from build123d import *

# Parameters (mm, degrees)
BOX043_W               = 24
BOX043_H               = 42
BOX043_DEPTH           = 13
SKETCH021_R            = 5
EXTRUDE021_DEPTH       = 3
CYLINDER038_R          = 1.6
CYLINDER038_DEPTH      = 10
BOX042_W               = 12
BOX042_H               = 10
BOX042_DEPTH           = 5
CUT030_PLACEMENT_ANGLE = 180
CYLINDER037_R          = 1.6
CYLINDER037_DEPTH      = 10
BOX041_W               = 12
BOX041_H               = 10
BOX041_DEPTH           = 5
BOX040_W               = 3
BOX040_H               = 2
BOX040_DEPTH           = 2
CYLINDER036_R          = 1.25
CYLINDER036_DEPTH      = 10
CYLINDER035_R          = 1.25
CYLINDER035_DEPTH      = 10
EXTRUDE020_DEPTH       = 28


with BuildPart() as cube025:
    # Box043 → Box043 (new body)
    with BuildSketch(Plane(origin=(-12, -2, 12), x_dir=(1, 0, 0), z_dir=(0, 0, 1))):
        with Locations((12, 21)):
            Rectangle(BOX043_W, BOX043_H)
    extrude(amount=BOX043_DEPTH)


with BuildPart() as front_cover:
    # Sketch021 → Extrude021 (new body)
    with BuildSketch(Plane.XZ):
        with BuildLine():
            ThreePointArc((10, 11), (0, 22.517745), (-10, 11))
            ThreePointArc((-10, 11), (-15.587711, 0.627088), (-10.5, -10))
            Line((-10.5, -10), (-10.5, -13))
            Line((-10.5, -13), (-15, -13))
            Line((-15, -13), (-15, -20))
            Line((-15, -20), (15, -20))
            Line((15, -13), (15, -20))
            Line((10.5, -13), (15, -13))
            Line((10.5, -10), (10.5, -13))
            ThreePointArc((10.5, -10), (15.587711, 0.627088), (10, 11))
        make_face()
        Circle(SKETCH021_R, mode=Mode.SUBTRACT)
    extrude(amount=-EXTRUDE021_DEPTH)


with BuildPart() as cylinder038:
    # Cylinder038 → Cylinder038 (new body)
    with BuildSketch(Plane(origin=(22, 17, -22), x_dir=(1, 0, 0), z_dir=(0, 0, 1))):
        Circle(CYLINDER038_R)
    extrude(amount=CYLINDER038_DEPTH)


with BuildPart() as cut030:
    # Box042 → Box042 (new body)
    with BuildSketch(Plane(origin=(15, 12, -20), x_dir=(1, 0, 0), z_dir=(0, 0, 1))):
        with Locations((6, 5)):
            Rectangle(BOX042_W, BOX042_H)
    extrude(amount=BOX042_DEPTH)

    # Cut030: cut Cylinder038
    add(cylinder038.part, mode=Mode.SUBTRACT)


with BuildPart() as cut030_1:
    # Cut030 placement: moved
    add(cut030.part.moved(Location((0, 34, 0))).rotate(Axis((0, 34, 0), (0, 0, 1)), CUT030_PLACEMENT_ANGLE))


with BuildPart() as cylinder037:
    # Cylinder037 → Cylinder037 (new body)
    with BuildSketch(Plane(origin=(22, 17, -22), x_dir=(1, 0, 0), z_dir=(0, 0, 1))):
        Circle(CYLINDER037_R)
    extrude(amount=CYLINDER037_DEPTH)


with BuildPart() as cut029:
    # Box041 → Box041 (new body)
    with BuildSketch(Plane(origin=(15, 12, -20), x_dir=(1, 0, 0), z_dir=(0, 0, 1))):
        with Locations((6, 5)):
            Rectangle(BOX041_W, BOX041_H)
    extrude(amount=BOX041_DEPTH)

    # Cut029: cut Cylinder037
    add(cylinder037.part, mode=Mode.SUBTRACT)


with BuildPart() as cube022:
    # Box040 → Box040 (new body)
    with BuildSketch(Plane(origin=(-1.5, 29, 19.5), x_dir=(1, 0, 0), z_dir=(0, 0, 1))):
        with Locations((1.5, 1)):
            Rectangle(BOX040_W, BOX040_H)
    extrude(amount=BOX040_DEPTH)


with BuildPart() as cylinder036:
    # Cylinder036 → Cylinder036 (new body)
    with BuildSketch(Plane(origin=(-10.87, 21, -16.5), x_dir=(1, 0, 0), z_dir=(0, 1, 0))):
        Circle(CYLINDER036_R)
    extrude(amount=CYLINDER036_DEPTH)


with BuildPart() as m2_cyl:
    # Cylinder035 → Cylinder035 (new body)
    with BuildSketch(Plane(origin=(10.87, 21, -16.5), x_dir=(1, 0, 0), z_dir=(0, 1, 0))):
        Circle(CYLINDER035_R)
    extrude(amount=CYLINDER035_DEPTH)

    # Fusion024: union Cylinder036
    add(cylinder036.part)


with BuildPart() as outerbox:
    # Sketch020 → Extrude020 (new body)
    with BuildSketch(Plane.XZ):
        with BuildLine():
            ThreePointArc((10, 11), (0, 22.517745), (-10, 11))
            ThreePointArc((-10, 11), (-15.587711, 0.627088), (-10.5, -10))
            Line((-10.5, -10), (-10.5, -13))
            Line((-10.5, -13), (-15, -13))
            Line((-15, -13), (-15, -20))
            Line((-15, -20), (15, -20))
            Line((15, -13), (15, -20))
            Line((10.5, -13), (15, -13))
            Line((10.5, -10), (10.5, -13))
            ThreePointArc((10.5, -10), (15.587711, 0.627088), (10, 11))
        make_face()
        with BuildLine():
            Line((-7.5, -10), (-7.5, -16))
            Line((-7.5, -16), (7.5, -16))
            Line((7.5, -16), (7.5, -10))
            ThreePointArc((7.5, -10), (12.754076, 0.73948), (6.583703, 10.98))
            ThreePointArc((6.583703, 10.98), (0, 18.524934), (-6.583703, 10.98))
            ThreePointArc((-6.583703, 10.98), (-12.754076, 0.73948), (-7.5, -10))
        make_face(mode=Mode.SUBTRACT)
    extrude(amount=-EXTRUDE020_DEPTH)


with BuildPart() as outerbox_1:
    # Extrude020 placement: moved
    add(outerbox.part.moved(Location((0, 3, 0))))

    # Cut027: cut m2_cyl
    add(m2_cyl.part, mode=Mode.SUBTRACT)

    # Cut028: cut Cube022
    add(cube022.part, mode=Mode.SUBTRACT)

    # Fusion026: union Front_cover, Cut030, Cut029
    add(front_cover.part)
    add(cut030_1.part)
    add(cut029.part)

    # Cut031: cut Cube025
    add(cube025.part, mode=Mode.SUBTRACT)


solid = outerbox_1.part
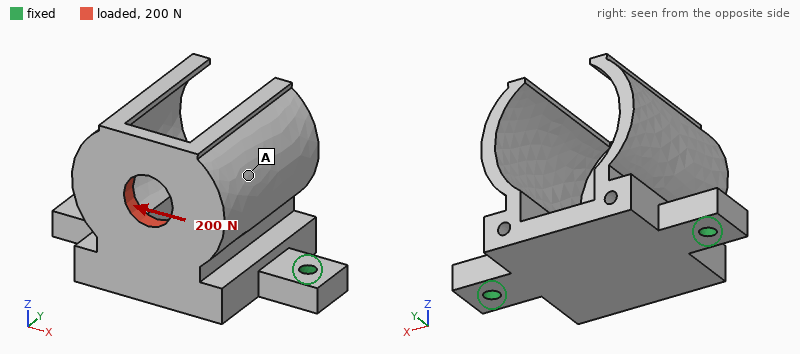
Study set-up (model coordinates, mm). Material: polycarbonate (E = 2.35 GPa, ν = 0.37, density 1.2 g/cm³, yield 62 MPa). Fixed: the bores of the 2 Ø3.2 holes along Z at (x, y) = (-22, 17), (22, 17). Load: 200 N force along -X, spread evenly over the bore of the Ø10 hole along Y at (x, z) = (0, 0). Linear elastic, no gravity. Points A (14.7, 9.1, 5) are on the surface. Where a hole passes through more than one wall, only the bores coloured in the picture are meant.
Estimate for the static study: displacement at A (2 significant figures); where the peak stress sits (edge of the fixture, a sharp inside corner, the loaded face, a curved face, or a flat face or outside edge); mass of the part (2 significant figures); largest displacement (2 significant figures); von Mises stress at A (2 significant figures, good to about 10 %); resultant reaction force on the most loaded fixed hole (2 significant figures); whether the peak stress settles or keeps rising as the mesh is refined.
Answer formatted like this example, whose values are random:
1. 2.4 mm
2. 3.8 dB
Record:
1. 0.52 mm
2. edge of the fixture
3. 15 g
4. 0.67 mm
5. 2.2 MPa
6. 160 N
7. keeps rising
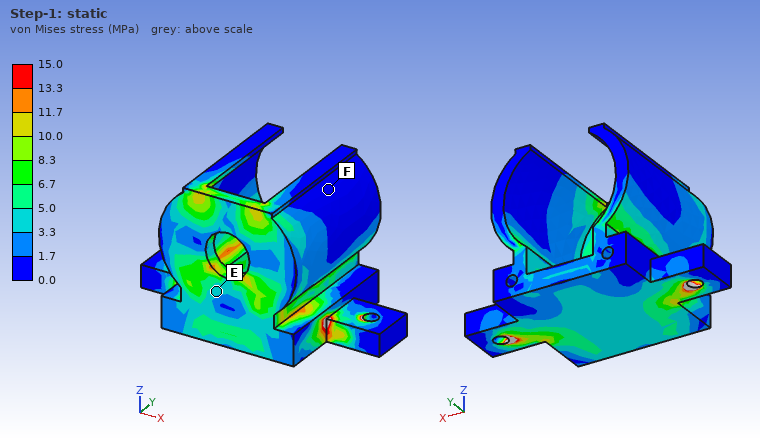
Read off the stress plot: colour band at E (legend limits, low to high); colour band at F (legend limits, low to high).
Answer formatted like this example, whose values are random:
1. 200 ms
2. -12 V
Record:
1. 3.3 to 5.0 MPa
2. 0.0 to 1.7 MPa
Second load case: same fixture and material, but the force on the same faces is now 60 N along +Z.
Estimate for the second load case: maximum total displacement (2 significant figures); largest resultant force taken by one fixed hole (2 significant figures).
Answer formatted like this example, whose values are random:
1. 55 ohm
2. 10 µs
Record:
1. 0.53 mm
2. 30 N
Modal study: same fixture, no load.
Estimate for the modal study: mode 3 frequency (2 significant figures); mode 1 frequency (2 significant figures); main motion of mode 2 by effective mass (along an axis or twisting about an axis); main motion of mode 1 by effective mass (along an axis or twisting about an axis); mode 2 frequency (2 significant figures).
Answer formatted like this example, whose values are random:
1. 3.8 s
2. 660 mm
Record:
1. 1200 Hz
2. 630 Hz
3. along X
4. along Y
5. 1100 Hz
